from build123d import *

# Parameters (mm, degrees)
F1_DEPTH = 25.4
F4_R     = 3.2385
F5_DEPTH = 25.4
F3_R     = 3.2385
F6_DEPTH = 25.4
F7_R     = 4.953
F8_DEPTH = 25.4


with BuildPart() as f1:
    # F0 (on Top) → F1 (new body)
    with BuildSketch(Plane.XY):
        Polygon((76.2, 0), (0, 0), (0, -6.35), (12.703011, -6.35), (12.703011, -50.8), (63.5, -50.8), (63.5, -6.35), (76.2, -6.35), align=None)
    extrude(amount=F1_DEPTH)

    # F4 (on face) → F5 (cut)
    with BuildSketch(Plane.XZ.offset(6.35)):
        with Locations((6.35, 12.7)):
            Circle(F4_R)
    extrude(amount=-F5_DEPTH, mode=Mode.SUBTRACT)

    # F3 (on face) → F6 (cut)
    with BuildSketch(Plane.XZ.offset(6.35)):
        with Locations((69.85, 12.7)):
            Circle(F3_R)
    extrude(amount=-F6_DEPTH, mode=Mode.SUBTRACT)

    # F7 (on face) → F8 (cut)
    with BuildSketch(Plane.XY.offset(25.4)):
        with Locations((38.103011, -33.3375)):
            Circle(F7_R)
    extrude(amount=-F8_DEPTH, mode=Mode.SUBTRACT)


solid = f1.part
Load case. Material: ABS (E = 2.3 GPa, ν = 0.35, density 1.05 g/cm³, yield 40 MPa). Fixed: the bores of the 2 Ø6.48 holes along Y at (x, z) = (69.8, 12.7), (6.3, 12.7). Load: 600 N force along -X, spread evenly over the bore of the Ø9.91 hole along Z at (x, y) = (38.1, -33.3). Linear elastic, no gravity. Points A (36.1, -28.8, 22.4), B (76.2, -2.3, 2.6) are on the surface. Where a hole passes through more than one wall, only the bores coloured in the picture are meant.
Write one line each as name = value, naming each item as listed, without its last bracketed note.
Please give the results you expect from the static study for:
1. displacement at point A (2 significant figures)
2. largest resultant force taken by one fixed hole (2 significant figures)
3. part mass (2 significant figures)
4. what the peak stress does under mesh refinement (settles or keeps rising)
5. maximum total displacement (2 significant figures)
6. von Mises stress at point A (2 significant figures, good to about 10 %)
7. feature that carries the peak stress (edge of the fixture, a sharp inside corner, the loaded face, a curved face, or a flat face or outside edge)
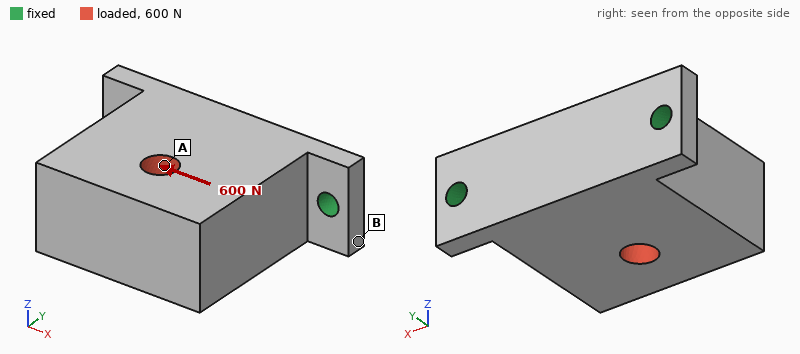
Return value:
displacement at point A = 0.064 mm
largest resultant force taken by one fixed hole = 440 N
part mass = 71 g
what the peak stress does under mesh refinement = keeps rising
maximum total displacement = 0.12 mm
von Mises stress at point A = 1.9 MPa
feature that carries the peak stress = edge of the fixture
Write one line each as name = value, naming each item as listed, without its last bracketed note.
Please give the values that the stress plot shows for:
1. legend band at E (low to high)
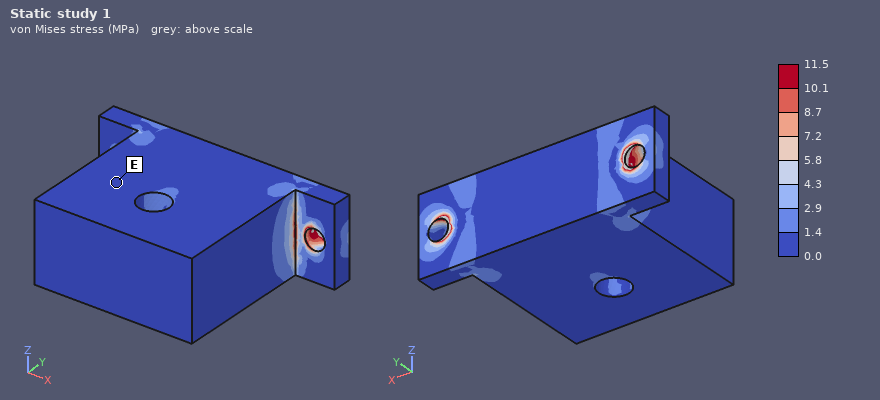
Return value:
legend band at E = 0.0 to 1.4 MPa
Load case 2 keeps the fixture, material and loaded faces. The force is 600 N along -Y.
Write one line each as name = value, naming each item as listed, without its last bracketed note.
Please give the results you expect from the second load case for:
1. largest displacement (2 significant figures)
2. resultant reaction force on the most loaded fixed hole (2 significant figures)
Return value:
largest displacement = 56 µm
resultant reaction force on the most loaded fixed hole = 330 N
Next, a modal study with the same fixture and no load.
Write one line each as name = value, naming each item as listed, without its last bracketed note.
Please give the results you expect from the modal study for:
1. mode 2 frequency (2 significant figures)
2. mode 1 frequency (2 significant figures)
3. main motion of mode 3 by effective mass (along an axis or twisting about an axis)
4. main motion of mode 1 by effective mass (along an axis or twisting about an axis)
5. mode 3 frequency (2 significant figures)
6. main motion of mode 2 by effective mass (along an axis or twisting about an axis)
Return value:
mode 2 frequency = 1900 Hz
mode 1 frequency = 490 Hz
main motion of mode 3 by effective mass = along Y
main motion of mode 1 by effective mass = along Z
mode 3 frequency = 2200 Hz
main motion of mode 2 by effective mass = along X
